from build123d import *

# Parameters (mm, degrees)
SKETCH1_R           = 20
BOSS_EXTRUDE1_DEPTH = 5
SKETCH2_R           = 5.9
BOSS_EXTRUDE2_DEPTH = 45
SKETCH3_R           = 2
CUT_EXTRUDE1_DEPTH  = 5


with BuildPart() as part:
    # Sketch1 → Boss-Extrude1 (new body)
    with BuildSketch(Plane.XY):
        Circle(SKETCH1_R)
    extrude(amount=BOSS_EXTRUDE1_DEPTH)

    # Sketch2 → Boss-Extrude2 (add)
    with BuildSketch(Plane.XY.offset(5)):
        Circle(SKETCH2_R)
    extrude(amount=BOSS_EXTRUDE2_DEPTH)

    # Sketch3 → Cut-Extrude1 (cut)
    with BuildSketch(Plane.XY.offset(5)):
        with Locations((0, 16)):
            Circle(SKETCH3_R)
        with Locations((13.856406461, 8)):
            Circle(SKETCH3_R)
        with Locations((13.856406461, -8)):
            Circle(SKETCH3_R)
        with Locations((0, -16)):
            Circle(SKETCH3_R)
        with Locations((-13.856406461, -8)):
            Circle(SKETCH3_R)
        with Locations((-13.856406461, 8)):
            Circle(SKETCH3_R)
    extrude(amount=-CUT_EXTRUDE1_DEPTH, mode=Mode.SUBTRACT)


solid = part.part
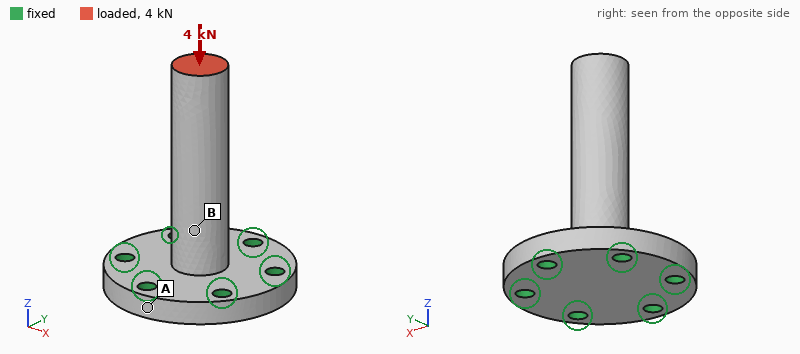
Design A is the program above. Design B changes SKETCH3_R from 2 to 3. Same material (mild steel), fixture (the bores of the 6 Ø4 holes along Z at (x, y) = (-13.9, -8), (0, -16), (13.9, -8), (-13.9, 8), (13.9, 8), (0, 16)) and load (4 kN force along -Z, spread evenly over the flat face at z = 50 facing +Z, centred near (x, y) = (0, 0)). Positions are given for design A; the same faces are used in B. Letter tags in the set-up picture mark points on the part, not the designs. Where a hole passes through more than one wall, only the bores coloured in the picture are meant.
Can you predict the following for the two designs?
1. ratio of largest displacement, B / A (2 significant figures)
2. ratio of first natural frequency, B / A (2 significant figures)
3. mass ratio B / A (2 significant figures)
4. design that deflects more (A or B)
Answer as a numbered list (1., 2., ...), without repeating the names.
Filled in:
1. 0.91
2. 1.0
3. 0.96
4. A
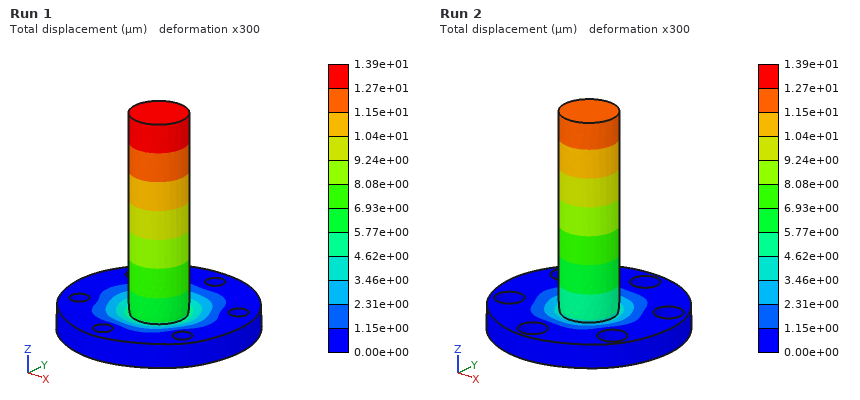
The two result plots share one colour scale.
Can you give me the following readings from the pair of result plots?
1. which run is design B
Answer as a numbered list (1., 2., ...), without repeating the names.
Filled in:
1. Run 2
